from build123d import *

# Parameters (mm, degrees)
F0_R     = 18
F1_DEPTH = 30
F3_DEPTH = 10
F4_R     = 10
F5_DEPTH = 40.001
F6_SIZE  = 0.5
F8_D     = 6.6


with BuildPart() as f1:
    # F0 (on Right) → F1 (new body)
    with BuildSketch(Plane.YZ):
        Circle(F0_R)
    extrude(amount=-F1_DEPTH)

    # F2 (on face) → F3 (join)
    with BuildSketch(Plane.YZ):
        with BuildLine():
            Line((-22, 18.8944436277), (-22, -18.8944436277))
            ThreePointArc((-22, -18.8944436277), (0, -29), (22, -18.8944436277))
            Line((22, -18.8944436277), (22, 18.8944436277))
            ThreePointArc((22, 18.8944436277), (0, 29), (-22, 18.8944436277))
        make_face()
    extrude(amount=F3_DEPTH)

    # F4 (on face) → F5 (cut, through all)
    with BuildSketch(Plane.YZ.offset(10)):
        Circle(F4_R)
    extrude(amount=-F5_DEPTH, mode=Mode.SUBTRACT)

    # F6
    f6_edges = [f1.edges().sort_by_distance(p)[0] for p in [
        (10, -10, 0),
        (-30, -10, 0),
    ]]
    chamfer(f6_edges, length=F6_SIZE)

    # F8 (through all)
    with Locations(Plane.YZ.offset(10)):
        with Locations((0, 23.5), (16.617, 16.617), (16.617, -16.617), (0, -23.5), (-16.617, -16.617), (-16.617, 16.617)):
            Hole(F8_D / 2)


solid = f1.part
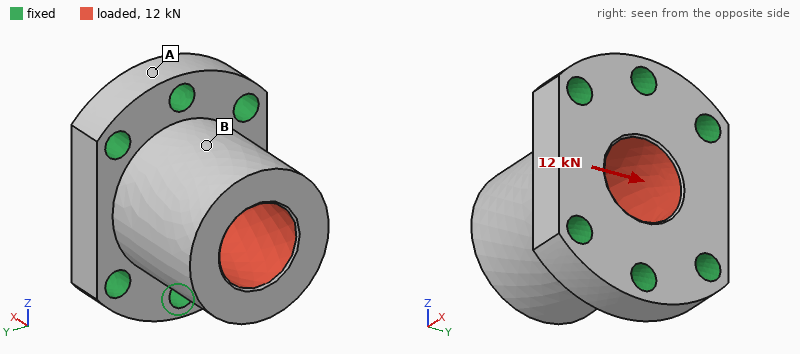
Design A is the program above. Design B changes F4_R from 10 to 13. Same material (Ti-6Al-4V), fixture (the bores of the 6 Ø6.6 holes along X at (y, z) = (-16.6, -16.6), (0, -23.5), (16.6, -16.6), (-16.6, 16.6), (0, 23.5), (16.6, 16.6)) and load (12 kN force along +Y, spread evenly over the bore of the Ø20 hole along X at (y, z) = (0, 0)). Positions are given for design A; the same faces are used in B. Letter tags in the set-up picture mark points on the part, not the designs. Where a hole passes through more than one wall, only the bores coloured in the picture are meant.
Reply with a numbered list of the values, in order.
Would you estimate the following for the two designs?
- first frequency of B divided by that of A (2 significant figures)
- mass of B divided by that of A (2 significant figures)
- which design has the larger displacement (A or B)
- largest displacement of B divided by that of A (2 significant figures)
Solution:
1. 1.0
2. 0.78
3. B
4. 1.3
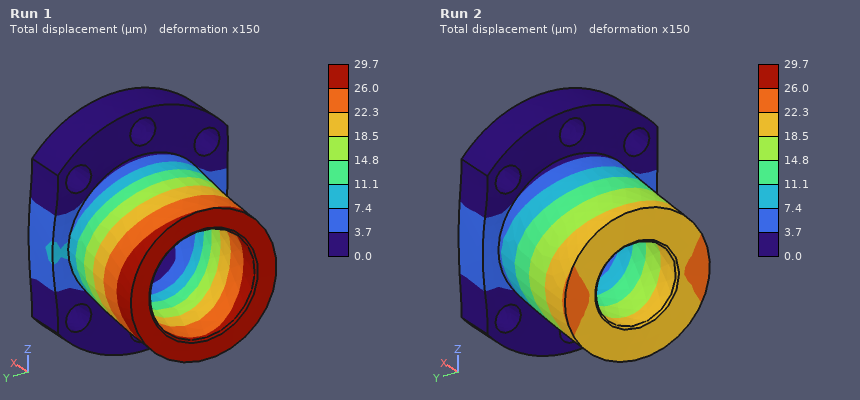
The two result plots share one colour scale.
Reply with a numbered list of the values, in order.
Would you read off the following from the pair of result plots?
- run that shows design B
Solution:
1. Run 1
